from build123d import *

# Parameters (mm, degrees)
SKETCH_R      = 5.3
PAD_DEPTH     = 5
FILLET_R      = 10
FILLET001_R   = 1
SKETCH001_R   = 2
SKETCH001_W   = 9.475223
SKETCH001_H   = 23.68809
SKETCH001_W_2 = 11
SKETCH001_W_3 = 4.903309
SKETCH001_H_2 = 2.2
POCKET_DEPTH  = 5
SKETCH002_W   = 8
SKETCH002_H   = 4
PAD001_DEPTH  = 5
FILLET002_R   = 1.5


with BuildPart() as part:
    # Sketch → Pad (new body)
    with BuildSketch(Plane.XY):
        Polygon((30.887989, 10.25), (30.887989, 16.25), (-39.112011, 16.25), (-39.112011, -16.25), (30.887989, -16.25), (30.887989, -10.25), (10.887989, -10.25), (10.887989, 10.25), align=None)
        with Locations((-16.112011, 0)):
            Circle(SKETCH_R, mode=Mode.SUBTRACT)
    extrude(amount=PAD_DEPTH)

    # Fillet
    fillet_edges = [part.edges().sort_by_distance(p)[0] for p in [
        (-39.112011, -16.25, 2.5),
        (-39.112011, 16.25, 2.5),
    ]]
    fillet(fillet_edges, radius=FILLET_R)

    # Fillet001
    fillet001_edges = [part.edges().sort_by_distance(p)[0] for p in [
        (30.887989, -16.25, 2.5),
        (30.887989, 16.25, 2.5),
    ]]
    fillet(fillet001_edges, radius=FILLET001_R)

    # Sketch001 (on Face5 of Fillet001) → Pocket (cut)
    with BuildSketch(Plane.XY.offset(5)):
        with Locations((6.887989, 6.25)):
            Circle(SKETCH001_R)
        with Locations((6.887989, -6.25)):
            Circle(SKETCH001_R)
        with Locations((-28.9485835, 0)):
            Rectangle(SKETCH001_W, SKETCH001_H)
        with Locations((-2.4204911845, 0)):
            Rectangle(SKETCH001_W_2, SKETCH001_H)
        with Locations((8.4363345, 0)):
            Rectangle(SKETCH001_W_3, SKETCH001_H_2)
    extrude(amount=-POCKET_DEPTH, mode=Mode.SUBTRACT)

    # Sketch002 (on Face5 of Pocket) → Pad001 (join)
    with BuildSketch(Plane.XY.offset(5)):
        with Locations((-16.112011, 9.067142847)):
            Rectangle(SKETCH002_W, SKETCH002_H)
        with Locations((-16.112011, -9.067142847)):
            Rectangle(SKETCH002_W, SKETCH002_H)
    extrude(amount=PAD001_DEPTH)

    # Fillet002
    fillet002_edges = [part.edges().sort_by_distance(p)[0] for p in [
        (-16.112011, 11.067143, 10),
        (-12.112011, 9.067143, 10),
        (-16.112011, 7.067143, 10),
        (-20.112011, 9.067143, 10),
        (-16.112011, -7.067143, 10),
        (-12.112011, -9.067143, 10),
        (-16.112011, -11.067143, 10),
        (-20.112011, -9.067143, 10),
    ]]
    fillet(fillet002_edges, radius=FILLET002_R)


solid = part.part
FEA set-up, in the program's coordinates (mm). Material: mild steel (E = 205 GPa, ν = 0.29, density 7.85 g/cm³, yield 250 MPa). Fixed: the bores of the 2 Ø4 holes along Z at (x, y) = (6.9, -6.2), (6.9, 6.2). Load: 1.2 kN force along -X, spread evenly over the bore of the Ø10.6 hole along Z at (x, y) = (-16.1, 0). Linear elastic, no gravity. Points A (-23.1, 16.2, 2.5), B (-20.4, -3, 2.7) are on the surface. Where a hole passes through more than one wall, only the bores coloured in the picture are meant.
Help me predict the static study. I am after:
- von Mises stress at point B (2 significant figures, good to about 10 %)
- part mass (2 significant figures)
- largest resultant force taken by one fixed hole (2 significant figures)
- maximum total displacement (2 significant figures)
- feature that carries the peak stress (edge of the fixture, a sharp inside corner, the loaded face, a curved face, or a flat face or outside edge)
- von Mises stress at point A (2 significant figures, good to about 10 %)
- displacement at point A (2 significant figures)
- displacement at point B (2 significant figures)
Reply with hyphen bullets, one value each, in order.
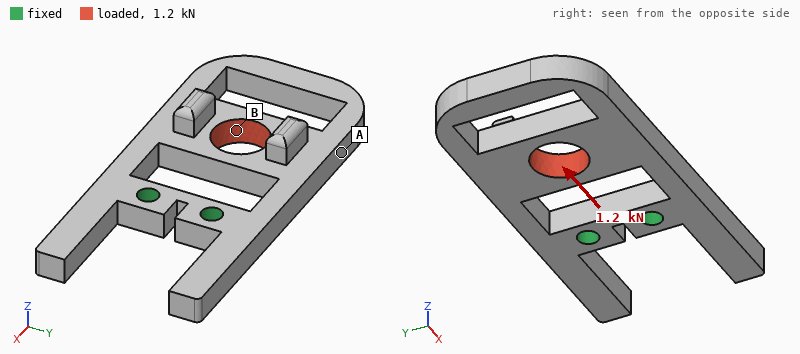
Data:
- 23 MPa
- 50 g
- 610 N
- 11 µm
- edge of the fixture
- 12 MPa
- 5.7 µm
- 7.9 µm
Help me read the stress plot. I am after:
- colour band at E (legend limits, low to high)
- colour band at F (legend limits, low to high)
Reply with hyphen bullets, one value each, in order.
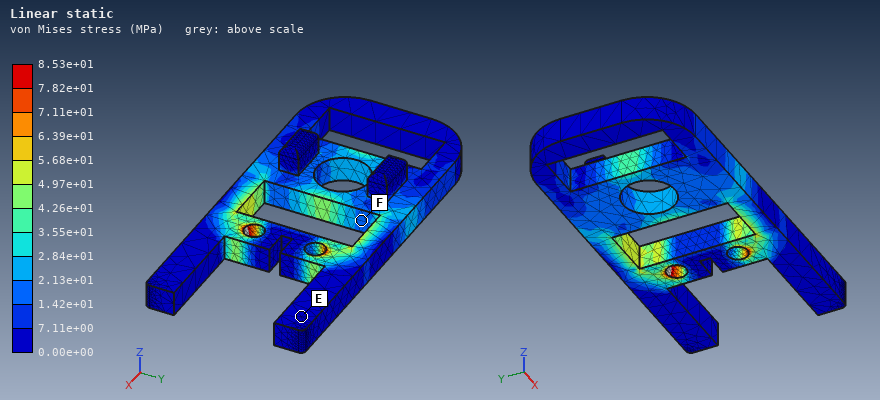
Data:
- 0.00e+00 to 7.11e+00 MPa
- 1.42e+01 to 2.13e+01 MPa
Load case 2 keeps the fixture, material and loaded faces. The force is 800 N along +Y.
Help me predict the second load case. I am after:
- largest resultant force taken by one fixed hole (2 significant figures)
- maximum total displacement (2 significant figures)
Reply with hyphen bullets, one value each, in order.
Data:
- 630 N
- 55 µm
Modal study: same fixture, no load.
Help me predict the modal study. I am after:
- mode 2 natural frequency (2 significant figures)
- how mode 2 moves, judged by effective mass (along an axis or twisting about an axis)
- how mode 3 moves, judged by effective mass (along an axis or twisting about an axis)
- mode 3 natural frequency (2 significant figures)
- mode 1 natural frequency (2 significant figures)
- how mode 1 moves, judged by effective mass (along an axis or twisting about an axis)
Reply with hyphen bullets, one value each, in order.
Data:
- 3600 Hz
- along Y
- twisting about X
- 4200 Hz
- 1300 Hz
- along Z
